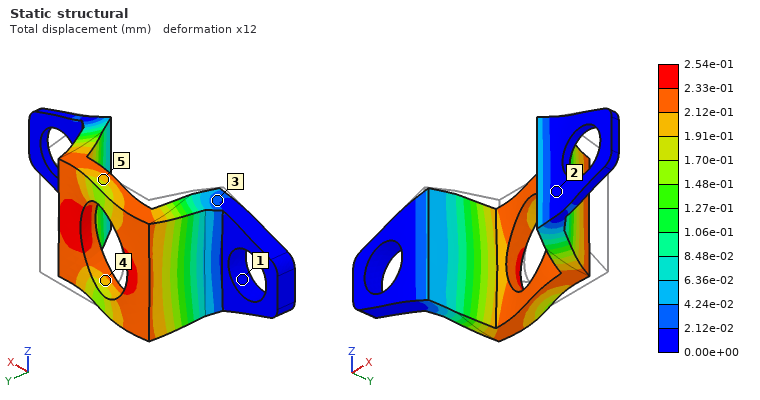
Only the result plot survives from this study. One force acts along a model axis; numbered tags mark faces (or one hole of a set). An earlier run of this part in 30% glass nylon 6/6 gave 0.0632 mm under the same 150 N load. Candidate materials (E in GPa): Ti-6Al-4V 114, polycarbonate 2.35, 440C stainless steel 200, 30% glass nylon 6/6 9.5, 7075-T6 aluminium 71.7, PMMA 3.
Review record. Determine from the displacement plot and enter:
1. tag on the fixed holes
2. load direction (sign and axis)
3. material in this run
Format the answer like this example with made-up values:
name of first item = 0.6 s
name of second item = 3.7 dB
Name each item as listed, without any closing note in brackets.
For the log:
tag on the fixed holes = 1
load direction = -X
material in this run = polycarbonate
